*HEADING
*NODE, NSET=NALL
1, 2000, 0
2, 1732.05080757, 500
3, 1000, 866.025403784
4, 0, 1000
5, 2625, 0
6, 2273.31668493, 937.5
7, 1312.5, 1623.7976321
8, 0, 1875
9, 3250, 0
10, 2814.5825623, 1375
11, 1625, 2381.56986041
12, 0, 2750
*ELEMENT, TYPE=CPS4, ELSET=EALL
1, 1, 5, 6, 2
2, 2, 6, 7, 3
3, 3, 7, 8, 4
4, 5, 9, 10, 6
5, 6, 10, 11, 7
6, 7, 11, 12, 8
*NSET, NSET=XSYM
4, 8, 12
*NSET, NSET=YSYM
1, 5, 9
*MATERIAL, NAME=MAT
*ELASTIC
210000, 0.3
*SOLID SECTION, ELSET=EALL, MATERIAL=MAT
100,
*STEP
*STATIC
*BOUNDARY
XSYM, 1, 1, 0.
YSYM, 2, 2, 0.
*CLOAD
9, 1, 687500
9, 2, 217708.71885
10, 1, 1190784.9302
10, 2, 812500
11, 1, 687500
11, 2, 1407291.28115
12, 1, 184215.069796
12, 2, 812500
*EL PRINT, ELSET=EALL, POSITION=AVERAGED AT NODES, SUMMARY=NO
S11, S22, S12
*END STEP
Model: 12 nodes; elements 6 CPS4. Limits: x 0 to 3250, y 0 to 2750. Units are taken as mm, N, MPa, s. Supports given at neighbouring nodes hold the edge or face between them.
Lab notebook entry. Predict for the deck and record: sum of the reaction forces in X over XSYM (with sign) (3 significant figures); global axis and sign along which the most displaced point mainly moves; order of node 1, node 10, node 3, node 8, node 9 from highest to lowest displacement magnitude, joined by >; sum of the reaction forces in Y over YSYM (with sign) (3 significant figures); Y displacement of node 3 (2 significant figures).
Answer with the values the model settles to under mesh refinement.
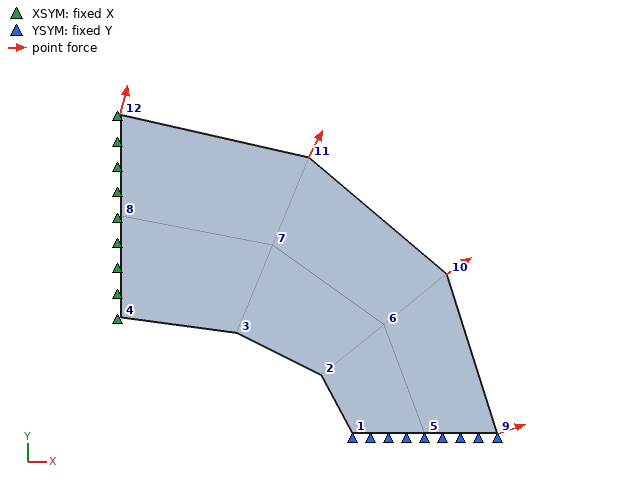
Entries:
-2.75e+06 N
+Y
node 8 > node 3 > node 10 > node 1 > node 9
-3.25e+06 N
0.43 mm
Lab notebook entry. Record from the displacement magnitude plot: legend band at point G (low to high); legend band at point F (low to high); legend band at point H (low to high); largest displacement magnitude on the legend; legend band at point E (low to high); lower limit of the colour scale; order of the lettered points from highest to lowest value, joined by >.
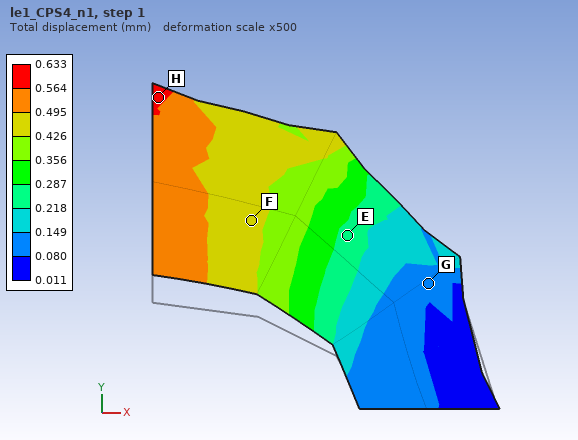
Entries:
0.080 to 0.149 mm
0.426 to 0.495 mm
0.564 to 0.633 mm
0.633 mm
0.218 to 0.287 mm
0.011 mm
H > F > E > G
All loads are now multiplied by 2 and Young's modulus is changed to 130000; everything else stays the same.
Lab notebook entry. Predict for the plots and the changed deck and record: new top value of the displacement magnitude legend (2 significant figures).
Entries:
2.0 mm
